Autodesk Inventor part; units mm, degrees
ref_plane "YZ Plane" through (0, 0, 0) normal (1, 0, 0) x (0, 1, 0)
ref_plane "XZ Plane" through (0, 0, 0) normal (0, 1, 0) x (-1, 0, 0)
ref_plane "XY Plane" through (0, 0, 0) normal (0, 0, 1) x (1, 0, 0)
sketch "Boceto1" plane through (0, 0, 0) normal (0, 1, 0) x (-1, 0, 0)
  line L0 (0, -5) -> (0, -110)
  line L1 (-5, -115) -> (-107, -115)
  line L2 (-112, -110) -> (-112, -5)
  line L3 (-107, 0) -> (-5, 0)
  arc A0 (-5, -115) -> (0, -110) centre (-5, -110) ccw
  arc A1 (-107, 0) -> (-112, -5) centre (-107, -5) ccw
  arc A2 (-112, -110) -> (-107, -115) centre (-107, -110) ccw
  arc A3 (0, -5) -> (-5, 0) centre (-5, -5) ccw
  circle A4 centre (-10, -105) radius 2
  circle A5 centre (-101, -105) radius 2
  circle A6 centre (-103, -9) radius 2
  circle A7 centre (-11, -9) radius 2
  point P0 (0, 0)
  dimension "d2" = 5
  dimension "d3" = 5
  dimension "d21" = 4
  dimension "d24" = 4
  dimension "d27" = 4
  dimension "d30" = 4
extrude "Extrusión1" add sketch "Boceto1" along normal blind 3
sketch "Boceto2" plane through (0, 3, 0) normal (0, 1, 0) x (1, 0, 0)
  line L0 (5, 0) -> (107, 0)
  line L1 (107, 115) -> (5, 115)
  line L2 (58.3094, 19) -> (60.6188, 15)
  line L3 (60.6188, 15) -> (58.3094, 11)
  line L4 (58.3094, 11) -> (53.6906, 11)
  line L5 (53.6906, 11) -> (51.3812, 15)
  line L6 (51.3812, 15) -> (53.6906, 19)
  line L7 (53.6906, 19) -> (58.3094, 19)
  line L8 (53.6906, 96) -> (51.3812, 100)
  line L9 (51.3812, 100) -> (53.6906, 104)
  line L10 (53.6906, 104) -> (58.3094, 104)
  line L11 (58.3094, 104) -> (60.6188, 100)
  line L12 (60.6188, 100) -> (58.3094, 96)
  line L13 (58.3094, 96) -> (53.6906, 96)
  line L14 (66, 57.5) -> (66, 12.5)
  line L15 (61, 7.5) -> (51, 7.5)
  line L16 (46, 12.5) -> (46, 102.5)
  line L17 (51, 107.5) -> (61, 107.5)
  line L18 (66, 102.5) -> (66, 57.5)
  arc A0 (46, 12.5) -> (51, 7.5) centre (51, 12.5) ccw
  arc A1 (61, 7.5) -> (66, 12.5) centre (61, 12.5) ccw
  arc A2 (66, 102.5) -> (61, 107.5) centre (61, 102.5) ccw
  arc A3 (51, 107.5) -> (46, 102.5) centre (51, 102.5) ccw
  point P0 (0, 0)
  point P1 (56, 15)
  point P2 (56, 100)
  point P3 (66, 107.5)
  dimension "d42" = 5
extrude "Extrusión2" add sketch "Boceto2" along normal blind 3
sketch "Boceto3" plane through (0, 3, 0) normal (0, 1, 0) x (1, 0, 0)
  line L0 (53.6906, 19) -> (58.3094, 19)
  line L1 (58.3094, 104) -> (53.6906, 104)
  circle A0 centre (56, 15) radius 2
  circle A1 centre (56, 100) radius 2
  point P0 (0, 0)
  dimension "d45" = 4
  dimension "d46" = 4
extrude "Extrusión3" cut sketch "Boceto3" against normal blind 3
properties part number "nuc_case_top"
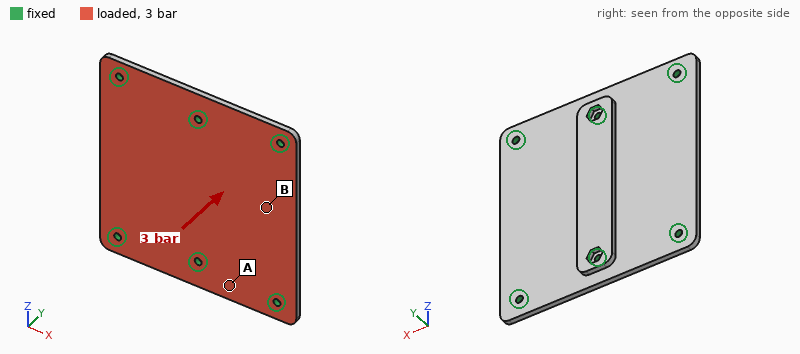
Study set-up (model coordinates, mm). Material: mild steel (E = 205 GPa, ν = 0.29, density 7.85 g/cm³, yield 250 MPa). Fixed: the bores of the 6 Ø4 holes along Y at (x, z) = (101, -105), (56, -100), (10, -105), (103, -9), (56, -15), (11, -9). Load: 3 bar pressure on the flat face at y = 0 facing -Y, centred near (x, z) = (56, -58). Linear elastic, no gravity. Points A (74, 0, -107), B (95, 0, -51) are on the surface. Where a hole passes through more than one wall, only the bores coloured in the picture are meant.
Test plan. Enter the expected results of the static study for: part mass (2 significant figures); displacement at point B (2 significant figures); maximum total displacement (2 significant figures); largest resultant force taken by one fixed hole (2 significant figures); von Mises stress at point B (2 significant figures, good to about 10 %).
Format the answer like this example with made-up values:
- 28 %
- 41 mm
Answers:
- 350 g
- 0.097 mm
- 0.13 mm
- 1.3 kN
- 45 MPa
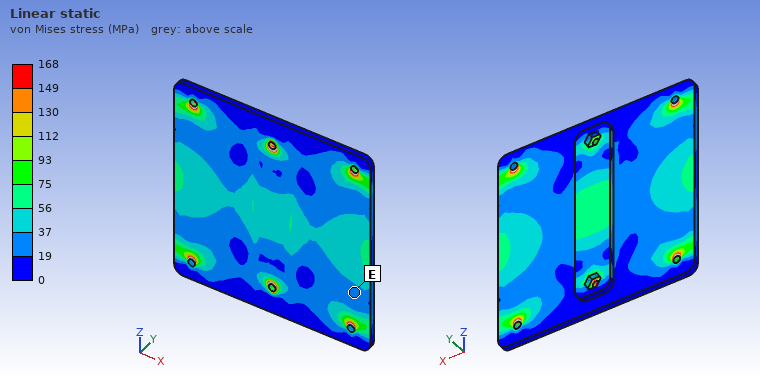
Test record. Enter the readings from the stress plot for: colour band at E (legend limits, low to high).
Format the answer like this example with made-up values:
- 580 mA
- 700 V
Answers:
- 19 to 37 MPa
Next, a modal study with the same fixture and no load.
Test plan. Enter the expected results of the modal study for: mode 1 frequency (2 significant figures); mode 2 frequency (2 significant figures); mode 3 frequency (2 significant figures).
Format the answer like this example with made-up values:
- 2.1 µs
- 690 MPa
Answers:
- 2000 Hz
- 2100 Hz
- 3400 Hz
